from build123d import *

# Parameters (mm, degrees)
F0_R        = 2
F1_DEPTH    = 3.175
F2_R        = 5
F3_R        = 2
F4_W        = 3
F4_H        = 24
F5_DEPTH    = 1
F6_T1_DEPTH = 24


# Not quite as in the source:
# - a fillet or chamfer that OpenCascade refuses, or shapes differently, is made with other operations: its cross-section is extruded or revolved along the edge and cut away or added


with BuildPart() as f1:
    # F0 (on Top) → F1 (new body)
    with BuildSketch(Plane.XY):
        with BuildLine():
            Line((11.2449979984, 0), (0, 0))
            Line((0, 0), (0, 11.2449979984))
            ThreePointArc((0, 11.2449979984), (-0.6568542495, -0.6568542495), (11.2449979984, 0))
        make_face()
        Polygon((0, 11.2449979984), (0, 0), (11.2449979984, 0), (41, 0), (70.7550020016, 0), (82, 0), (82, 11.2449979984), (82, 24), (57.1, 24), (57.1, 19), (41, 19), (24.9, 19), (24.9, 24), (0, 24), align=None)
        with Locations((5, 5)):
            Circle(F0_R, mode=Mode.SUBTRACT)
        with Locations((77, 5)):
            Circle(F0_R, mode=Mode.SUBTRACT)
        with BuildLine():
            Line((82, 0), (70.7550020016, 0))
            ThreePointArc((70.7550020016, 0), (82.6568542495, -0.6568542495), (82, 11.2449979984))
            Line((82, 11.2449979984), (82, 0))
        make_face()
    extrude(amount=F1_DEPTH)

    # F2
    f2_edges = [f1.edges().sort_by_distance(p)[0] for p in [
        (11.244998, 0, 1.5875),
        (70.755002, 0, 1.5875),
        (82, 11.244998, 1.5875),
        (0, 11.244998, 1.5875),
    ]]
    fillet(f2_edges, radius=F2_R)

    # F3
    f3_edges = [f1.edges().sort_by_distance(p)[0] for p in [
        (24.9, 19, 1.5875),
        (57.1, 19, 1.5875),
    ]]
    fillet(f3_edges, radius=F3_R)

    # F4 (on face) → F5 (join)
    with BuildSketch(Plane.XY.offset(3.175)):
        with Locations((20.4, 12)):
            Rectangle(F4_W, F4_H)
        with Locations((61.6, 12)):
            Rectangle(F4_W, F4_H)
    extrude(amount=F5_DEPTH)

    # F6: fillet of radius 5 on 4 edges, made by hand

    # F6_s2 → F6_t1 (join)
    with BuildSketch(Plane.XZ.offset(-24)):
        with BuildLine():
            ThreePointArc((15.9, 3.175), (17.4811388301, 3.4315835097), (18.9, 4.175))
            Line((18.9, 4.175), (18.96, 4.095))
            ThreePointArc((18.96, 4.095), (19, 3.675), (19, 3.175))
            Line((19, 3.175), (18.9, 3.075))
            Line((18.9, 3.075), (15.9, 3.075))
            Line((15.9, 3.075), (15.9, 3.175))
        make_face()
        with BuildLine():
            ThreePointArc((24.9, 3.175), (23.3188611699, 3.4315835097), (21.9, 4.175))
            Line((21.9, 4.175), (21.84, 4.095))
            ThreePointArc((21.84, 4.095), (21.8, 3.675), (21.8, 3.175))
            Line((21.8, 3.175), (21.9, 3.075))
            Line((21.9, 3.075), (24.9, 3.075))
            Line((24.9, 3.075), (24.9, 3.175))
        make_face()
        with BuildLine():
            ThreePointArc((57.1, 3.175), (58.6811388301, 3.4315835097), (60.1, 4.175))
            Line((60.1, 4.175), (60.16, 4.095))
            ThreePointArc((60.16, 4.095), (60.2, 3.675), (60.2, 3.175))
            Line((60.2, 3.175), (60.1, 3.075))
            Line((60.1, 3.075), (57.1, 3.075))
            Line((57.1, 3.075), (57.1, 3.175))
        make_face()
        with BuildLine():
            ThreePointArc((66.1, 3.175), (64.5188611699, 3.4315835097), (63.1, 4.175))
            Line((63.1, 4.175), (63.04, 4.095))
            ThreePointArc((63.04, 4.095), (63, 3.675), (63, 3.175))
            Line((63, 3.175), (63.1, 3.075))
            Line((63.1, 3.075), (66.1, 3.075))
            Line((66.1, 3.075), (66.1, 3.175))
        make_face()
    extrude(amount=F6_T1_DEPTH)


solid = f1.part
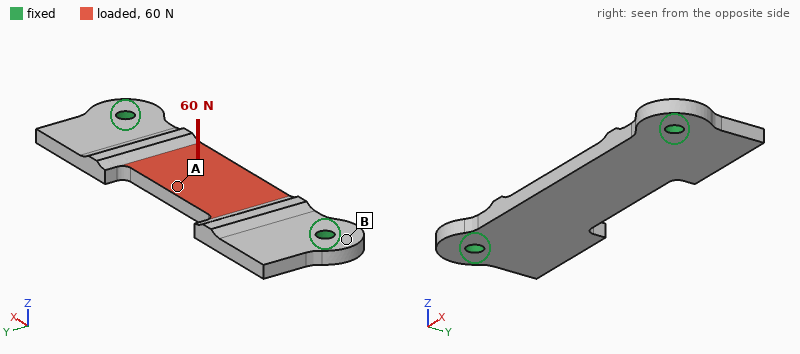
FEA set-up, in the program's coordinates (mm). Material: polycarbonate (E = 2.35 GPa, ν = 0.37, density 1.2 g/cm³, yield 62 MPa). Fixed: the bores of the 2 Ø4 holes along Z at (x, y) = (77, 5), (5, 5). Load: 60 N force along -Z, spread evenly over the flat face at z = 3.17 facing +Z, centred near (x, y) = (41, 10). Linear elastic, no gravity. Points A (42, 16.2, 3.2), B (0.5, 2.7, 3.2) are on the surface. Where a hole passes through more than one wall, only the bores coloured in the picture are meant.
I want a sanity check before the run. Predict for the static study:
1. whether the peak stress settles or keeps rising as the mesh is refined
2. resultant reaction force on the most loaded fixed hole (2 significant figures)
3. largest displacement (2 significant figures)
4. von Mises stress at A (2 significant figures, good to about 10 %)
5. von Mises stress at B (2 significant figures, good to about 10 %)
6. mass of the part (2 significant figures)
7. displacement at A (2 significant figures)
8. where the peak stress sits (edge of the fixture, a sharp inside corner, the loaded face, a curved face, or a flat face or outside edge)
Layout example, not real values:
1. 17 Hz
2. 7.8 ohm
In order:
1. keeps rising
2. 30 N
3. 0.91 mm
4. 9.8 MPa
5. 2.7 MPa
6. 7.5 g
7. 0.87 mm
8. edge of the fixture
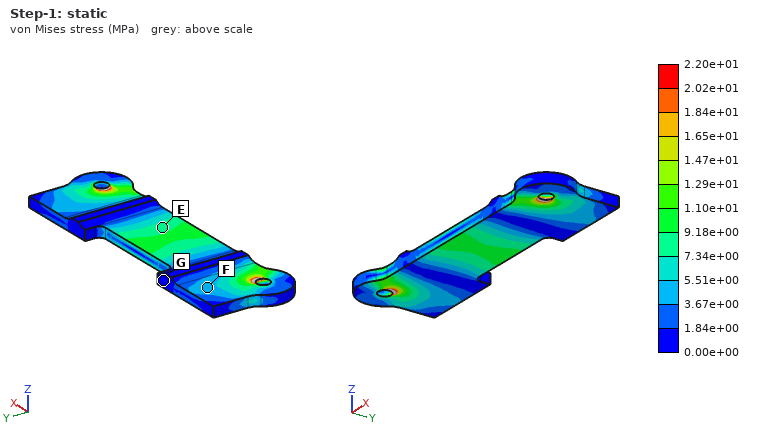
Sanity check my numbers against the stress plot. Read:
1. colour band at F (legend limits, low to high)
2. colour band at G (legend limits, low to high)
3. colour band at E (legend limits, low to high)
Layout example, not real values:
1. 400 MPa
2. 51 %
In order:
1. 3.67e+00 to 5.51e+00 MPa
2. 0.00e+00 to 1.84e+00 MPa
3. 7.34e+00 to 9.18e+00 MPa
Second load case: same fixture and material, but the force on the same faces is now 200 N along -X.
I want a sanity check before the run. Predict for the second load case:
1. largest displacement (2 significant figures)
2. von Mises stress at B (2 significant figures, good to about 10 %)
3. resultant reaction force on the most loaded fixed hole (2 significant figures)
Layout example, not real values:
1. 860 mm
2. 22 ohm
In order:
1. 51 µm
2. 0.97 MPa
3. 100 N
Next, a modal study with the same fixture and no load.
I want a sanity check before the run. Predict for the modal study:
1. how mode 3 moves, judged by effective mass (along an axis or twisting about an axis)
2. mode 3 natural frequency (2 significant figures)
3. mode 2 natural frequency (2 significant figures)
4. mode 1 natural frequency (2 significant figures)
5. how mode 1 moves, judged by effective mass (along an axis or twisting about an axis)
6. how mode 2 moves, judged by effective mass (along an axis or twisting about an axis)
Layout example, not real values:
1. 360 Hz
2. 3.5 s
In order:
1. twisting about Y
2. 1800 Hz
3. 1500 Hz
4. 820 Hz
5. along Z
6. twisting about X
